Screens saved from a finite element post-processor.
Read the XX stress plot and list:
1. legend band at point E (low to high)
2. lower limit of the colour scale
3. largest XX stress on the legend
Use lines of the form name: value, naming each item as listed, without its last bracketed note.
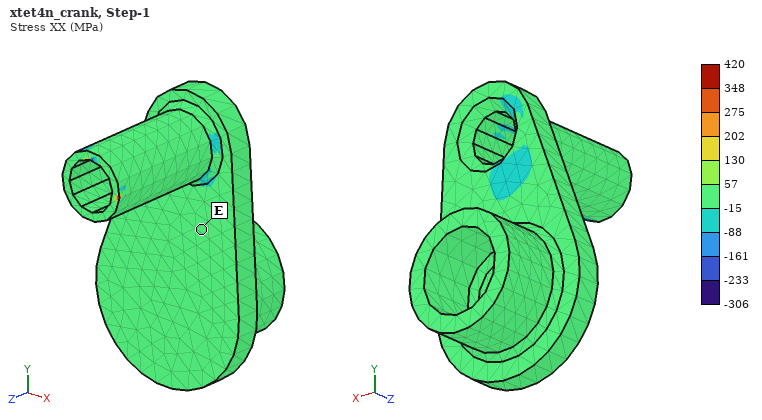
legend band at point E: -15 to 57 MPa
lower limit of the colour scale: -306 MPa
largest XX stress on the legend: 420 MPa
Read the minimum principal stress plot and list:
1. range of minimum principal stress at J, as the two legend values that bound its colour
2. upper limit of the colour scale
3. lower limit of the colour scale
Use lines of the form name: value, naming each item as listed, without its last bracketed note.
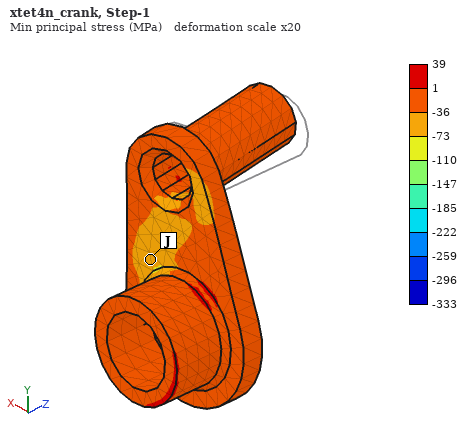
range of minimum principal stress at J, as the two legend values that bound its colour: -73 to -36 MPa
upper limit of the colour scale: 39 MPa
lower limit of the colour scale: -333 MPa
